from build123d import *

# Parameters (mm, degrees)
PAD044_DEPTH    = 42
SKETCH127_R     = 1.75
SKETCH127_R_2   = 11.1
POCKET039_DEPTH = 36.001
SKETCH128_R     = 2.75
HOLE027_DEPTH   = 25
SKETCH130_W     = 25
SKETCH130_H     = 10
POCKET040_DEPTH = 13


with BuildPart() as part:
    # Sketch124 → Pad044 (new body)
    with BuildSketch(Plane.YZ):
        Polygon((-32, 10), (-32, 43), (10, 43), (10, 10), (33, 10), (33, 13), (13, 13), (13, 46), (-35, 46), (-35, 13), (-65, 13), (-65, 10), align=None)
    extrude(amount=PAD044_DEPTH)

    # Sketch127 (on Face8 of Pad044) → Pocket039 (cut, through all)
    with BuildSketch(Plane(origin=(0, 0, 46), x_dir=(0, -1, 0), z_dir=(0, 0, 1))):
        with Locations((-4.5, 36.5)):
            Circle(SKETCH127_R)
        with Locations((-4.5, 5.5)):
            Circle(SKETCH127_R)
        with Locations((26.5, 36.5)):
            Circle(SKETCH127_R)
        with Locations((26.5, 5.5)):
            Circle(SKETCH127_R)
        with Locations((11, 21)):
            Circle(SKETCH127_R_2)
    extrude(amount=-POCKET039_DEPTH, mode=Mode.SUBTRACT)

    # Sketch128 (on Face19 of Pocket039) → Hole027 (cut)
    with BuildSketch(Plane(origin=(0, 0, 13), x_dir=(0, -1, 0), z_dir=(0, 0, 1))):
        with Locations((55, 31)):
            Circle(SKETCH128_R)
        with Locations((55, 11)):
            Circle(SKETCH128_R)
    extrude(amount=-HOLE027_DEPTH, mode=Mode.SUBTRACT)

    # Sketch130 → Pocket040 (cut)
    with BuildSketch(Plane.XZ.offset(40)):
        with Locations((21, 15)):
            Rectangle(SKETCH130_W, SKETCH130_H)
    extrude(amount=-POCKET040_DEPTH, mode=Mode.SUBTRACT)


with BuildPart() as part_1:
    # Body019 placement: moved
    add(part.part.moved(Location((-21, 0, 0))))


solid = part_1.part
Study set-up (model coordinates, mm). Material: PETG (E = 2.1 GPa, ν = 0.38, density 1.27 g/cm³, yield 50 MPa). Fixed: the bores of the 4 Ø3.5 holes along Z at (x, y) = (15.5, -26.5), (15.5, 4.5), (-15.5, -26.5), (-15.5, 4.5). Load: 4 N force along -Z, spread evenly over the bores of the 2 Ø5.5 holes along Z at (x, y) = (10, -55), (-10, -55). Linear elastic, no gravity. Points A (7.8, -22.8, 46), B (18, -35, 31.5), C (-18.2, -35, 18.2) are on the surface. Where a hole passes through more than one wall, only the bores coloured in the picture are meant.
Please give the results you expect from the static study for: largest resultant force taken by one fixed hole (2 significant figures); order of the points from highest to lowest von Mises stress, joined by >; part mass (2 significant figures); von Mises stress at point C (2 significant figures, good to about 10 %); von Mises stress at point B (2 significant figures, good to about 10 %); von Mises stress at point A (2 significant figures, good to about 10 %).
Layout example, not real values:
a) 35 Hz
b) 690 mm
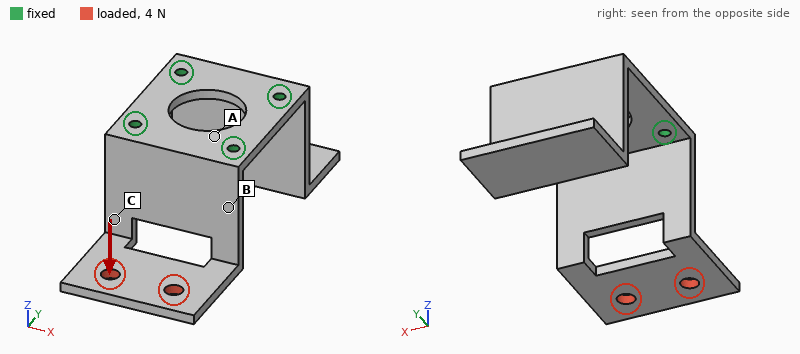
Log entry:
a) 2.3 N
b) C > B > A
c) 23 g
d) 3.2 MPa
e) 1.7 MPa
f) 0.52 MPa
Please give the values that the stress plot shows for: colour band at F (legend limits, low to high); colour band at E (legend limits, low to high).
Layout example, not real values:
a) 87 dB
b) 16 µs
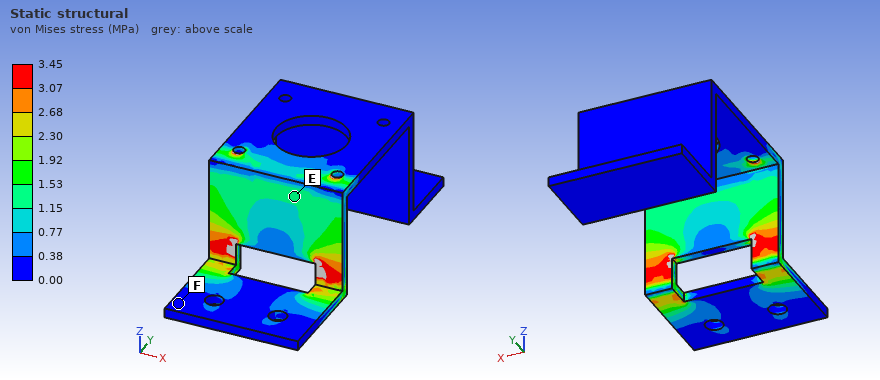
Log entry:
a) 0.00 to 0.38 MPa
b) 1.15 to 1.53 MPa
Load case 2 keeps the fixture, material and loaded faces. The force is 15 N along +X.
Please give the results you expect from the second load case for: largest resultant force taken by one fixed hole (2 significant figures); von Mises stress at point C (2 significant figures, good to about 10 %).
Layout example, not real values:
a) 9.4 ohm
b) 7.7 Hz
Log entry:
a) 21 N
b) 4.6 MPa
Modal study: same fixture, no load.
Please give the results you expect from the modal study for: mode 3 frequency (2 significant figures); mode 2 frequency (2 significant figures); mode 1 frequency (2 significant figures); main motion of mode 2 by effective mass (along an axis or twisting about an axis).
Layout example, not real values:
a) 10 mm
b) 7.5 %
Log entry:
a) 340 Hz
b) 220 Hz
c) 160 Hz
d) along Y
